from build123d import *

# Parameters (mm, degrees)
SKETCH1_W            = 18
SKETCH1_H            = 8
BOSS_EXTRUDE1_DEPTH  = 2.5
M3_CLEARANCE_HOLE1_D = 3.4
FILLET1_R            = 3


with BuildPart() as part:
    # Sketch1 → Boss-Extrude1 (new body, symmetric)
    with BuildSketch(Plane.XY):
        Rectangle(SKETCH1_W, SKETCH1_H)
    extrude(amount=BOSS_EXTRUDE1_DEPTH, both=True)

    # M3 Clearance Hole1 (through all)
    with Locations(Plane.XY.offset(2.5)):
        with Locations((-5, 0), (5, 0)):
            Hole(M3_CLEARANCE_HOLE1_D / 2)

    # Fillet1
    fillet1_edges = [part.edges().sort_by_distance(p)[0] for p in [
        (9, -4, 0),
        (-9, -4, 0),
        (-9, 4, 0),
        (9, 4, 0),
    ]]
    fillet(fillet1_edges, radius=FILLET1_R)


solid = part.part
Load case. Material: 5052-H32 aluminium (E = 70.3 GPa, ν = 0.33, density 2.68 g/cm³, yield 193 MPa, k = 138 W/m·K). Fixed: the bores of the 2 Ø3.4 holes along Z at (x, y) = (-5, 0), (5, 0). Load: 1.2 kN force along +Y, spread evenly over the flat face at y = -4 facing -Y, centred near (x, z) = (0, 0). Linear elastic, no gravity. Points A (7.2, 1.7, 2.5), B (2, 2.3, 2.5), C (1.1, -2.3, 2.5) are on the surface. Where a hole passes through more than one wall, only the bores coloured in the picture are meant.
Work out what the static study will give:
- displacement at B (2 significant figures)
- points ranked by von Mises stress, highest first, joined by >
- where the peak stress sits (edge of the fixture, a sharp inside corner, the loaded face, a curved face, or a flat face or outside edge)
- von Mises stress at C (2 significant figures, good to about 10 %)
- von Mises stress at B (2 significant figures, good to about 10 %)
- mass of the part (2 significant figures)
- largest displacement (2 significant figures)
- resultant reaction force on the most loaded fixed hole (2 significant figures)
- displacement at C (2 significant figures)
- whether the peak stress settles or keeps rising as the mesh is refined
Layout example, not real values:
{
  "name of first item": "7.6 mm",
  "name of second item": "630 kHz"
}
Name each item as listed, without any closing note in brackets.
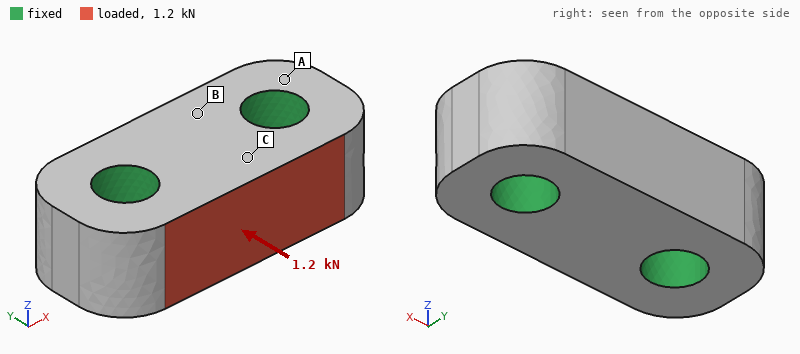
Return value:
{
  "displacement at B": "0.56 µm",
  "points ranked by von Mises stress, highest first, joined by >": "C > B > A",
  "where the peak stress sits": "edge of the fixture",
  "von Mises stress at C": "16 MPa",
  "von Mises stress at B": "9.8 MPa",
  "mass of the part": "1.6 g",
  "largest displacement": "1.8 µm",
  "resultant reaction force on the most loaded fixed hole": "620 N",
  "displacement at C": "1.3 µm",
  "whether the peak stress settles or keeps rising as the mesh is refined": "keeps rising"
}
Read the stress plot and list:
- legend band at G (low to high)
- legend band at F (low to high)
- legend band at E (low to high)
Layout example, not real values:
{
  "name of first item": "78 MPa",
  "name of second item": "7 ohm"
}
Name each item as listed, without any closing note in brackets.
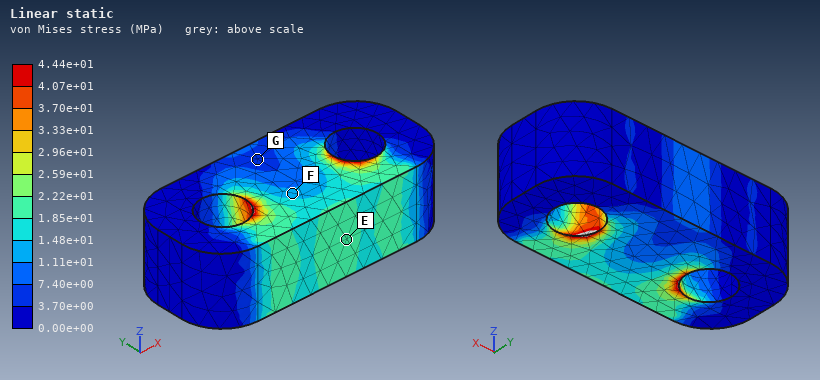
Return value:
{
  "legend band at G": "3.70e+00 to 7.40e+00 MPa",
  "legend band at F": "1.11e+01 to 1.48e+01 MPa",
  "legend band at E": "1.85e+01 to 2.22e+01 MPa"
}
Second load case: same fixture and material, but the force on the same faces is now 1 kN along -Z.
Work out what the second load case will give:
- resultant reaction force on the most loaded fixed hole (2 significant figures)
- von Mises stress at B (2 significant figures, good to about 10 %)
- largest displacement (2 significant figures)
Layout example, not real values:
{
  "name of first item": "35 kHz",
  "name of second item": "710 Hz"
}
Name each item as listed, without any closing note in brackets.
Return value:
{
  "resultant reaction force on the most loaded fixed hole": "500 N",
  "von Mises stress at B": "13 MPa",
  "largest displacement": "6.1 µm"
}
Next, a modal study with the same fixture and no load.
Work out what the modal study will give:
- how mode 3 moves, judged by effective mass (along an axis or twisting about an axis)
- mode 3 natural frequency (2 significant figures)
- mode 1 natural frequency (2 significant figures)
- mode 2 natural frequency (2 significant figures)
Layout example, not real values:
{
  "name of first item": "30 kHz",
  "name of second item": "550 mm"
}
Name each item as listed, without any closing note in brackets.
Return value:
{
  "how mode 3 moves, judged by effective mass": "along Y",
  "mode 3 natural frequency": "170 kHz",
  "mode 1 natural frequency": "150 kHz",
  "mode 2 natural frequency": "150 kHz"
}
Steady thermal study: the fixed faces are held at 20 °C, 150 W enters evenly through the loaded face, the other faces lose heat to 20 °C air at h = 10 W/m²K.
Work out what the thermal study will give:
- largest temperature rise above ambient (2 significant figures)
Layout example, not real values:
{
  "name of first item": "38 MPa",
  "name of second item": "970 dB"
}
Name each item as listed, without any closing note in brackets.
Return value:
{
  "largest temperature rise above ambient": "68 K"
}
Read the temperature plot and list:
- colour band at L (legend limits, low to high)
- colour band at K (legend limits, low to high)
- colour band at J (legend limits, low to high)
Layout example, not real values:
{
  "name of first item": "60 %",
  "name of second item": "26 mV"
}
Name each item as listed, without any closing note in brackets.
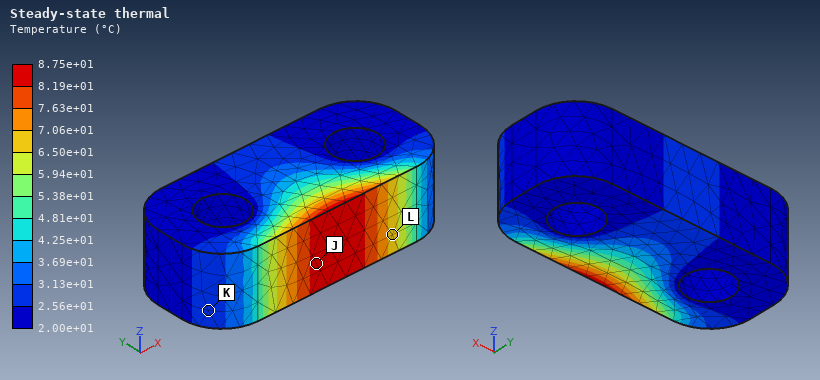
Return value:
{
  "colour band at L": "6.50e+01 to 7.06e+01 °C",
  "colour band at K": "2.56e+01 to 3.13e+01 °C",
  "colour band at J": "8.19e+01 to 8.75e+01 °C"
}
